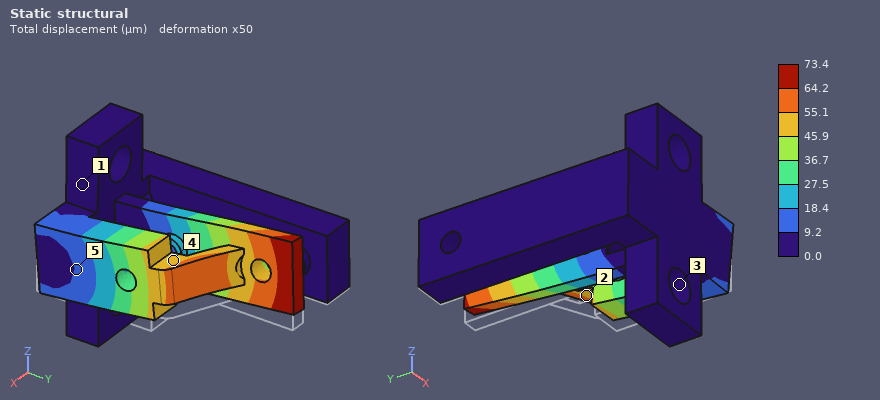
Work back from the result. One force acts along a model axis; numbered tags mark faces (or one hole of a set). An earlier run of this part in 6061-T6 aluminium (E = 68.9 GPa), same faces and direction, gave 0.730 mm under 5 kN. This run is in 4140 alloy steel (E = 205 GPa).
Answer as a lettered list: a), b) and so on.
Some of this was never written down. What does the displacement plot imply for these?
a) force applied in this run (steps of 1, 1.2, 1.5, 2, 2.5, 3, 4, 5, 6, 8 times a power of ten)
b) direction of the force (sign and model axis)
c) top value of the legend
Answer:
a) 1.5 kN
b) +Z
c) 73.4 µm
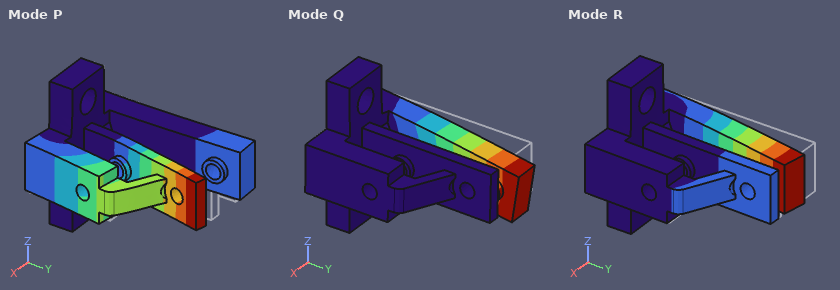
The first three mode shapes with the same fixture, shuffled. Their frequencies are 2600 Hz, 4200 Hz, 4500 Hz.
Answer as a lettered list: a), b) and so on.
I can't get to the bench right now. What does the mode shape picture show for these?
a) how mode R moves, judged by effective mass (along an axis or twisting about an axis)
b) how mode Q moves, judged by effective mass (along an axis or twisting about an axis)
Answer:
a) along X
b) along Z
